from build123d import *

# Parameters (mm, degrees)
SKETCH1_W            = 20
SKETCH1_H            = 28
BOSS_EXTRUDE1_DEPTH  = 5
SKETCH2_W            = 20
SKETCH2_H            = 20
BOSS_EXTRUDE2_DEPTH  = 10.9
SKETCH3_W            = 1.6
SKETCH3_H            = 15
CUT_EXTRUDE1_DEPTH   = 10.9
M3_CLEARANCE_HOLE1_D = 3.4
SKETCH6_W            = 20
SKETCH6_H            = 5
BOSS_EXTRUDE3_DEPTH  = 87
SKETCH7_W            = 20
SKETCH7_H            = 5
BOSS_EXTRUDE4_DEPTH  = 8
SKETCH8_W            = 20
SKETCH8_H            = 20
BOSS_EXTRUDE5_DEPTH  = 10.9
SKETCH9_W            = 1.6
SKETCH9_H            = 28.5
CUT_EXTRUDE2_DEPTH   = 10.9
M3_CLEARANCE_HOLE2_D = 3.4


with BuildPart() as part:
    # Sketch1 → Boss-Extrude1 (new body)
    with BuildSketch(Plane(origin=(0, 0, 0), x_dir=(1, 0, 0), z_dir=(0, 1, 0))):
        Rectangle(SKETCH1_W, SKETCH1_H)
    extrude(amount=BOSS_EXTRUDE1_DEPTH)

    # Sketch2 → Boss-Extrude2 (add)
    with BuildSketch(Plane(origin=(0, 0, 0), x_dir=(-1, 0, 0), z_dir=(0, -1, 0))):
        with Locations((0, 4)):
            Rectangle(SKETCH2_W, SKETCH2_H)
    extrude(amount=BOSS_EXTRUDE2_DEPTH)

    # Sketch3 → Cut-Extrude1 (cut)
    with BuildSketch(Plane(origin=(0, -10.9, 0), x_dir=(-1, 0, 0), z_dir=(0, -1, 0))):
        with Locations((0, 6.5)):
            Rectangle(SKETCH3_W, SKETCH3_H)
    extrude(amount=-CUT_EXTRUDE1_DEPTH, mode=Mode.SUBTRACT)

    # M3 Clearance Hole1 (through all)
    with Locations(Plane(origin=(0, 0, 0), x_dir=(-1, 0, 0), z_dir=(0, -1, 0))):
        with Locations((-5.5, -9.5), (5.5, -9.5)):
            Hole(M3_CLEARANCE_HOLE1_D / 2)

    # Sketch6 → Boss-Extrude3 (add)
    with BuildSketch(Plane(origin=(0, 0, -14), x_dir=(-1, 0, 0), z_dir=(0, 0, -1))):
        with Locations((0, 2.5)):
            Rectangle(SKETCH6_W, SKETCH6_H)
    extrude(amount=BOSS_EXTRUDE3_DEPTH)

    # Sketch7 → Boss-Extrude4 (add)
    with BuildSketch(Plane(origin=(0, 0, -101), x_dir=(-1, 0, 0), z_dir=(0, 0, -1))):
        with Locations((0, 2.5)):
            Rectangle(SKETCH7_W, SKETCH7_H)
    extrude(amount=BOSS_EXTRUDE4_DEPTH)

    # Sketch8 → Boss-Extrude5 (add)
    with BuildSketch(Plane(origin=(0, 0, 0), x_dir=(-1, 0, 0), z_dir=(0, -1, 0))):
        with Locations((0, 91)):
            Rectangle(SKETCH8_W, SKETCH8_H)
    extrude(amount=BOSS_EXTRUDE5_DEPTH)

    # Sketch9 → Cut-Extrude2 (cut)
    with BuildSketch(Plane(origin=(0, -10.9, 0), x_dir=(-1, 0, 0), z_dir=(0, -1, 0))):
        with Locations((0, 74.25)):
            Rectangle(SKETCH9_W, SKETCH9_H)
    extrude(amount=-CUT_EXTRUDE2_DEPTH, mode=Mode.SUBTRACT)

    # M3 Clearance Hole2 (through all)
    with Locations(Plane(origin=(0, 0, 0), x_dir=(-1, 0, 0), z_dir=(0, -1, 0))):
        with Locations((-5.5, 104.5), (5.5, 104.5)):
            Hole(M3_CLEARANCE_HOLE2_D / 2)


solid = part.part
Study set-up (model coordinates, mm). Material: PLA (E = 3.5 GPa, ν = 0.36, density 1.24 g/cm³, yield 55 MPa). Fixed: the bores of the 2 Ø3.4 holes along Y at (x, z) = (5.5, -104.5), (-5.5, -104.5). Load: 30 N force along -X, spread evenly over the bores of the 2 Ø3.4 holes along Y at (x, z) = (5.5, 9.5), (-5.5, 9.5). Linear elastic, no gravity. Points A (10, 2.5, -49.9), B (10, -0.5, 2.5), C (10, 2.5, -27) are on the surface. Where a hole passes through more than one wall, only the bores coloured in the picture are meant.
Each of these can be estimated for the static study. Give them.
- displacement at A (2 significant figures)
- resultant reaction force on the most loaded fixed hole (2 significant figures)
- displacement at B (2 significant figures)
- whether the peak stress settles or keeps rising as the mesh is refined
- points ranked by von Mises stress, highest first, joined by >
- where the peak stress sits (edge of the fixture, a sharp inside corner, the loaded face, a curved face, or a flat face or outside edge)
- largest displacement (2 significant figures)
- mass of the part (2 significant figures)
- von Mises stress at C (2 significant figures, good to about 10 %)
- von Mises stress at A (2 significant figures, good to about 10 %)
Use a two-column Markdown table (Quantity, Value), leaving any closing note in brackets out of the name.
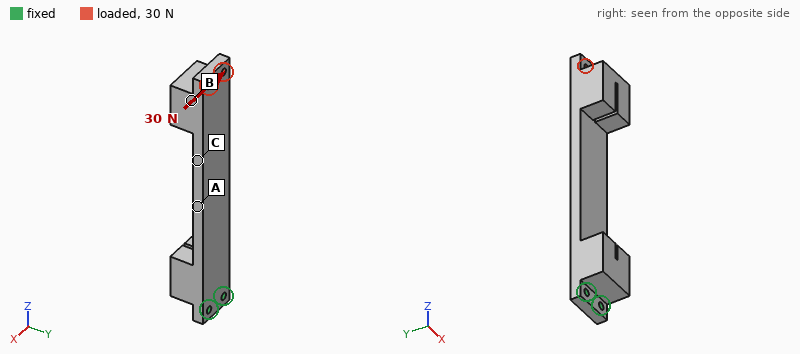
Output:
| Quantity | Value |
|---|---|
| displacement at A | 0.35 mm |
| resultant reaction force on the most loaded fixed hole | 270 N |
| displacement at B | 1.1 mm |
| whether the peak stress settles or keeps rising as the mesh is refined | keeps rising |
| points ranked by von Mises stress, highest first, joined by > | A > C > B |
| where the peak stress sits | edge of the fixture |
| largest displacement | 1.2 mm |
| mass of the part | 25 g |
| von Mises stress at C | 3.3 MPa |
| von Mises stress at A | 5.4 MPa |
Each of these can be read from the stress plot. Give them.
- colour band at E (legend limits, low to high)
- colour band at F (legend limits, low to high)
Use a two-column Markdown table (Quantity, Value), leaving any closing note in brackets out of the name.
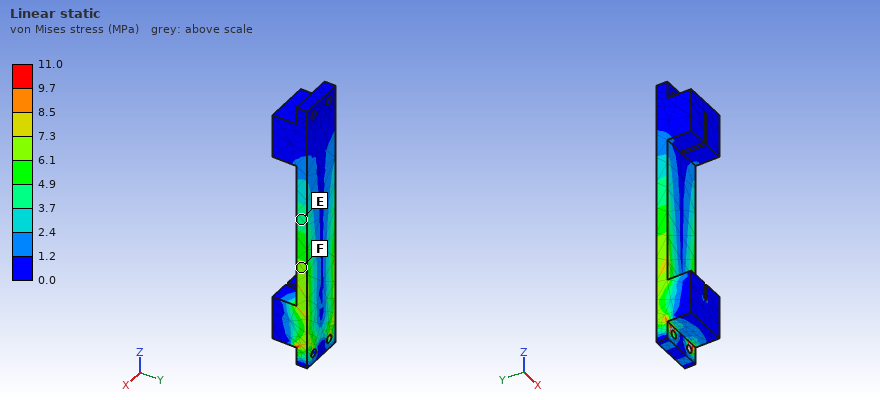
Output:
| Quantity | Value |
|---|---|
| colour band at E | 3.7 to 4.9 MPa |
| colour band at F | 6.1 to 7.3 MPa |
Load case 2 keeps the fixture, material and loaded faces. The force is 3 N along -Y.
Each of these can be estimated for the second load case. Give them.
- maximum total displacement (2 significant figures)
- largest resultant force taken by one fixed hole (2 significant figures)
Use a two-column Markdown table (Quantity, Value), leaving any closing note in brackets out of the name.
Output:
| Quantity | Value |
|---|---|
| maximum total displacement | 1.5 mm |
| largest resultant force taken by one fixed hole | 1.5 N |
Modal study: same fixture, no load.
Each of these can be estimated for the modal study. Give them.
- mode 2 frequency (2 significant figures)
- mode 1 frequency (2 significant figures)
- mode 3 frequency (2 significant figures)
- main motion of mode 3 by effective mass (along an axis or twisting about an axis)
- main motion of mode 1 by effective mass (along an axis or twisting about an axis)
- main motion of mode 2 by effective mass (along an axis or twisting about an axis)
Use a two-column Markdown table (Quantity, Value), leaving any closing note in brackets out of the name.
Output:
| Quantity | Value |
|---|---|
| mode 2 frequency | 290 Hz |
| mode 1 frequency | 89 Hz |
| mode 3 frequency | 600 Hz |
| main motion of mode 3 by effective mass | along Y |
| main motion of mode 1 by effective mass | along Y |
| main motion of mode 2 by effective mass | along X |
